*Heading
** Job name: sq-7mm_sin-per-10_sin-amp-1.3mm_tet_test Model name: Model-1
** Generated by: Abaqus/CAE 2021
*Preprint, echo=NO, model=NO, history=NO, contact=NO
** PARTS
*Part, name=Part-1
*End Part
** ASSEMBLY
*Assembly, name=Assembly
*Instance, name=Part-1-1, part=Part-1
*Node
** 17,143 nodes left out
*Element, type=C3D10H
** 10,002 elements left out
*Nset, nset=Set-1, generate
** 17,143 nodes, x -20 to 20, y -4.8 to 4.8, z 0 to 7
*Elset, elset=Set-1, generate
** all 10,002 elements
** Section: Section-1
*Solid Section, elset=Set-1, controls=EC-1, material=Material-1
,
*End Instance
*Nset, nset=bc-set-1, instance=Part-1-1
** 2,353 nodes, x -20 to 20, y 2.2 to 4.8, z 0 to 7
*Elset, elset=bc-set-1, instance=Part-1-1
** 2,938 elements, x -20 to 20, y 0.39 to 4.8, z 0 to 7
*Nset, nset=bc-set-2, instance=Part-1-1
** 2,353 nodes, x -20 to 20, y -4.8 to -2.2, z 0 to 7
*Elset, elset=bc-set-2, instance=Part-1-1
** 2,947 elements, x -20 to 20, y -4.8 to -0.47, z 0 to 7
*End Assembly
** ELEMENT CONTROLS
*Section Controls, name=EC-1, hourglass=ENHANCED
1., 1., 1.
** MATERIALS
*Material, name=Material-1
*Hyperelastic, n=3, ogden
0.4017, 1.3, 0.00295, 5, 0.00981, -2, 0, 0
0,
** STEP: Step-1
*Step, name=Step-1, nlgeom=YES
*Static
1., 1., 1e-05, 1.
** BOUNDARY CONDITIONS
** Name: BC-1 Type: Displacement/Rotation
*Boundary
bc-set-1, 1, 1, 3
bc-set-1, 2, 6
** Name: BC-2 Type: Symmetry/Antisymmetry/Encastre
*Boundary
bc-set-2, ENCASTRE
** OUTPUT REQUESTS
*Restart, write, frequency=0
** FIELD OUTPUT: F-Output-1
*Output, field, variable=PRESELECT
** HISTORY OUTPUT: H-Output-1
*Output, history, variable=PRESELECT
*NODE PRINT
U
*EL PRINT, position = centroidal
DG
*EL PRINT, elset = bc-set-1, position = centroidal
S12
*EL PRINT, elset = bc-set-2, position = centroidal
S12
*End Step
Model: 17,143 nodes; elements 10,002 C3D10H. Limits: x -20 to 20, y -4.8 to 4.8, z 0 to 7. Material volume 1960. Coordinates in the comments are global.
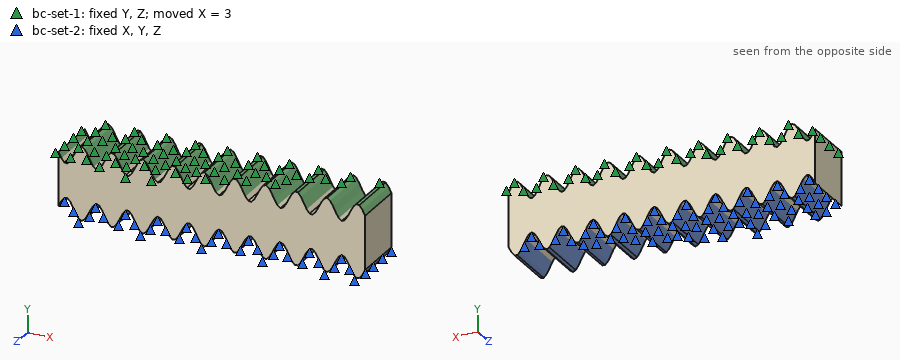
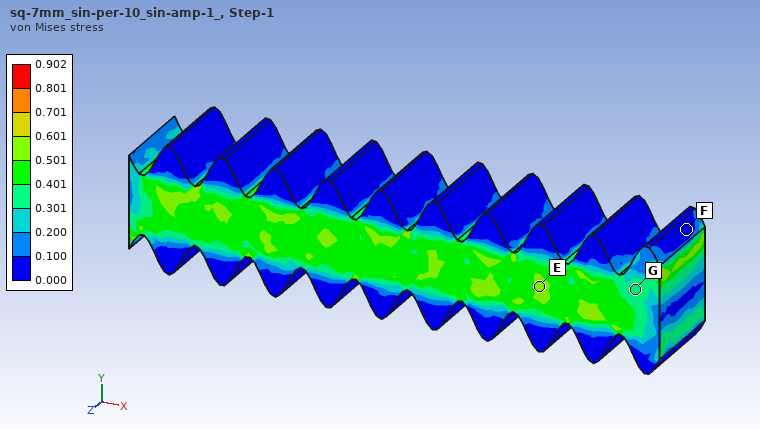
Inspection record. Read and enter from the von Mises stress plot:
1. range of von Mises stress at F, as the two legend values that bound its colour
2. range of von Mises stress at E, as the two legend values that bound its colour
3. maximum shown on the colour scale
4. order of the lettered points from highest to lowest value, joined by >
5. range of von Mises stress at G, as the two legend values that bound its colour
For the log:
0.000 to 0.100
0.501 to 0.601
0.902
E > G > F
0.301 to 0.401
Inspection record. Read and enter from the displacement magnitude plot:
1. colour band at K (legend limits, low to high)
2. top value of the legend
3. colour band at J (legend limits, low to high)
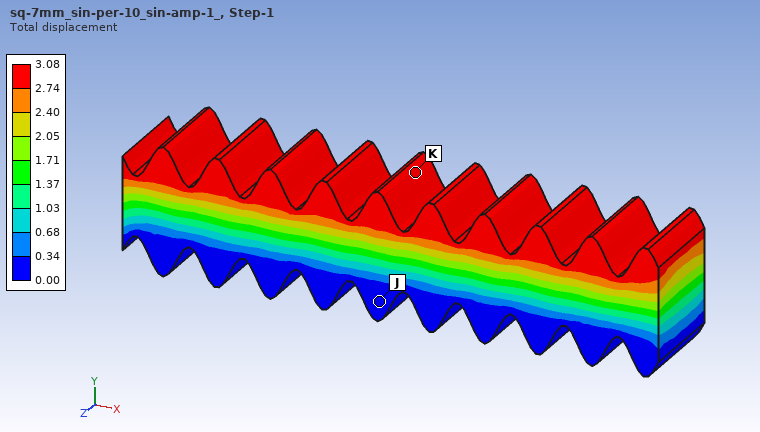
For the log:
2.74 to 3.08
3.08
0.00 to 0.34
